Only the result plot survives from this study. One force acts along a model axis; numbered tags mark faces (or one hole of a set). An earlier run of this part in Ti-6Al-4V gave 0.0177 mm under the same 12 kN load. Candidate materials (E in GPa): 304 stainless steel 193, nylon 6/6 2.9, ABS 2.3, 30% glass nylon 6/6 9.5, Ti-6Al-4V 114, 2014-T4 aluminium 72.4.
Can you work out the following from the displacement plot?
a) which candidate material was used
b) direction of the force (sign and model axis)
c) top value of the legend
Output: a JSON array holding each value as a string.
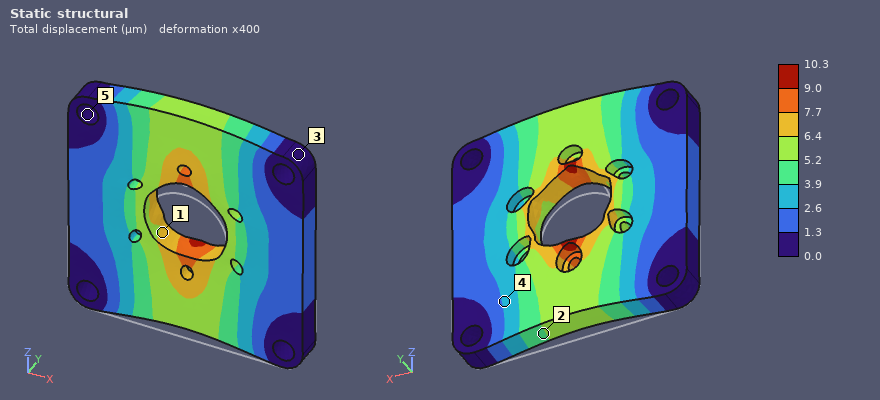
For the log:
["304 stainless steel", "+Z", "10.3 µm"]
